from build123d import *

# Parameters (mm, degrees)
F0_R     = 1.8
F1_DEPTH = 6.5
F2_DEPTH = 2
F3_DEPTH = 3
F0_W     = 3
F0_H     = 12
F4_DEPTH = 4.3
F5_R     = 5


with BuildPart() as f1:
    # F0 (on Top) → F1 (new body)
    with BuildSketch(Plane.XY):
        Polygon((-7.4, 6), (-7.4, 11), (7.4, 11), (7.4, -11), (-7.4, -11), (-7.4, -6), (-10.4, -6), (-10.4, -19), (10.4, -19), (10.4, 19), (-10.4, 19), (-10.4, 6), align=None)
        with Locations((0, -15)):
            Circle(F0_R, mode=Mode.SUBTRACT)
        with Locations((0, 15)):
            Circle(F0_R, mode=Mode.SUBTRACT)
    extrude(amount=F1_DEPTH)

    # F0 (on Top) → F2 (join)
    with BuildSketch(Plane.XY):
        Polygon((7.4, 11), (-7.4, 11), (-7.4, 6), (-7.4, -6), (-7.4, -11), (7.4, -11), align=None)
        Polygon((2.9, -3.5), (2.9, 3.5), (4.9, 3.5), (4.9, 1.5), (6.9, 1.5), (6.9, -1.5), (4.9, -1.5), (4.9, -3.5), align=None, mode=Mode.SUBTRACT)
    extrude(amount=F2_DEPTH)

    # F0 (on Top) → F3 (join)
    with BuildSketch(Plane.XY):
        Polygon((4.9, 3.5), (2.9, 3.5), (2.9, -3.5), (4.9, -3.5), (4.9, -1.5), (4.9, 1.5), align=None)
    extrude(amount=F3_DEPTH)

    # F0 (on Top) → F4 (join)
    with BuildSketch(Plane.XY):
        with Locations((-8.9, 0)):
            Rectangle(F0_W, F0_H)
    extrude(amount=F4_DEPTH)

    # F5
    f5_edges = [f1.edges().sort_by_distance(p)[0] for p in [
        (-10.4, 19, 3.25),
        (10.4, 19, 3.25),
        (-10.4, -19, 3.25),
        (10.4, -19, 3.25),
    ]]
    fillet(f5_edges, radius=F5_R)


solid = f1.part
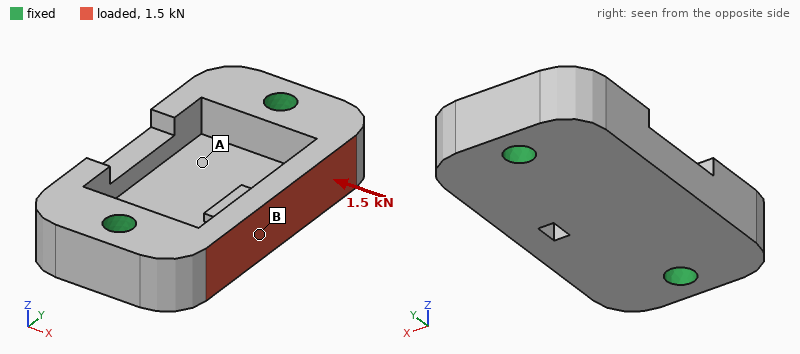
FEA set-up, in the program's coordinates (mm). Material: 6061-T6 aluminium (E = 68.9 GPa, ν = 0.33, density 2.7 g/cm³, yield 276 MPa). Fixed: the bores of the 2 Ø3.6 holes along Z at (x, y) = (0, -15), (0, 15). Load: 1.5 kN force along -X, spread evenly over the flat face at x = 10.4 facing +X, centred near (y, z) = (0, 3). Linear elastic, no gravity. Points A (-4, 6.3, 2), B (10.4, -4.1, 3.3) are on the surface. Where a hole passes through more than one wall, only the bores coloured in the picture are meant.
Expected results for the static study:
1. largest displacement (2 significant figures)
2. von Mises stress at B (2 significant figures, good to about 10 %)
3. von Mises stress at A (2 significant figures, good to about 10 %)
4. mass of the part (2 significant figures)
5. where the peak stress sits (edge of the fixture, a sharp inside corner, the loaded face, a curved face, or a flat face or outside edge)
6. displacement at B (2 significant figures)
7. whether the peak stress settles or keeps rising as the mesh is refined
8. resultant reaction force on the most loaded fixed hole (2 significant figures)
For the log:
30 µm
46 MPa
12 MPa
9.0 g
a sharp inside corner
17 µm
keeps rising
780 N
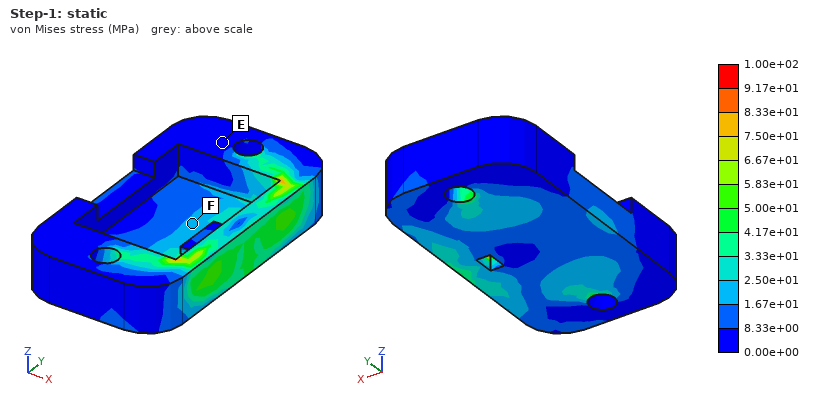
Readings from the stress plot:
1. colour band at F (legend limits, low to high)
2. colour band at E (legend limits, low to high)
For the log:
1.67e+01 to 2.50e+01 MPa
0.00e+00 to 8.33e+00 MPa
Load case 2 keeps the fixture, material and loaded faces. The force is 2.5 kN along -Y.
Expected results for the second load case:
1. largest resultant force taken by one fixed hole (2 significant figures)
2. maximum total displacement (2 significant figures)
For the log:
1.4 kN
15 µm
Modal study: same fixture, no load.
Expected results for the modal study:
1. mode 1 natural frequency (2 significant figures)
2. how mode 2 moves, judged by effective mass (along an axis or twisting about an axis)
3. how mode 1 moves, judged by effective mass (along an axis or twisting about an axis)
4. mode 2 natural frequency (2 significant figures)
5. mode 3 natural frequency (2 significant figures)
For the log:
21 kHz
twisting about Y
along Z
22 kHz
33 kHz
